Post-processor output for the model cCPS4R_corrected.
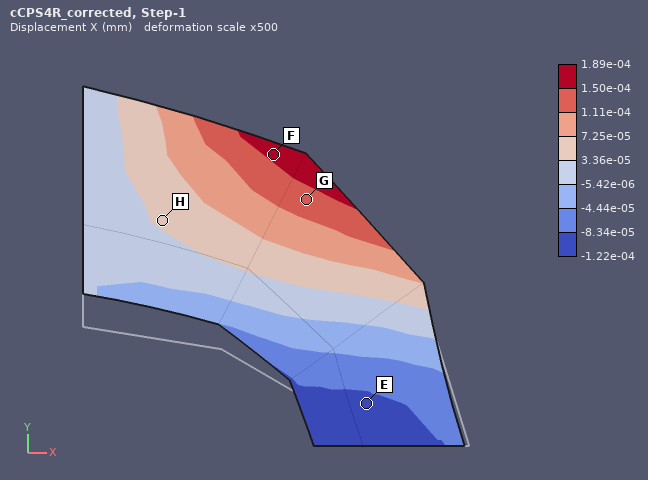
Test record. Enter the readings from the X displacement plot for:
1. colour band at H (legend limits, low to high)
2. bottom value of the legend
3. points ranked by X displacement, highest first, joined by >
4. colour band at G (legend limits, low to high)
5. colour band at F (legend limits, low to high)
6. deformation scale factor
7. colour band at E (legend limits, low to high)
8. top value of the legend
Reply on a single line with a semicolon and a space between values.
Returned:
3.36e-05 to 7.25e-05 mm; -1.22e-04 mm; F > G > H > E; 1.11e-04 to 1.50e-04 mm; 1.50e-04 to 1.89e-04 mm; 500; -1.22e-04 to -8.34e-05 mm; 1.89e-04 mm
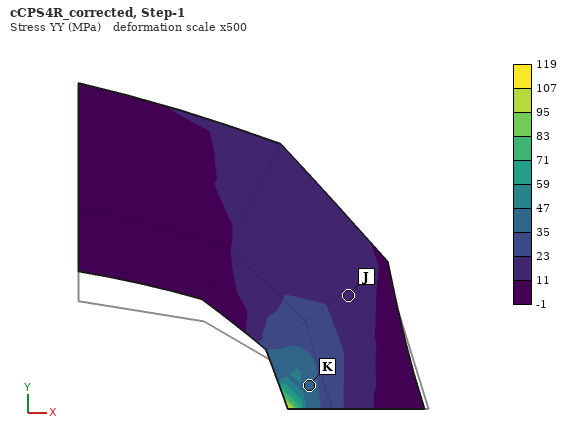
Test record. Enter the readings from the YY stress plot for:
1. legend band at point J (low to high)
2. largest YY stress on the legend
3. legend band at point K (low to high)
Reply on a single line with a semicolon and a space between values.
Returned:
11 to 23 MPa; 119 MPa; 35 to 47 MPa
